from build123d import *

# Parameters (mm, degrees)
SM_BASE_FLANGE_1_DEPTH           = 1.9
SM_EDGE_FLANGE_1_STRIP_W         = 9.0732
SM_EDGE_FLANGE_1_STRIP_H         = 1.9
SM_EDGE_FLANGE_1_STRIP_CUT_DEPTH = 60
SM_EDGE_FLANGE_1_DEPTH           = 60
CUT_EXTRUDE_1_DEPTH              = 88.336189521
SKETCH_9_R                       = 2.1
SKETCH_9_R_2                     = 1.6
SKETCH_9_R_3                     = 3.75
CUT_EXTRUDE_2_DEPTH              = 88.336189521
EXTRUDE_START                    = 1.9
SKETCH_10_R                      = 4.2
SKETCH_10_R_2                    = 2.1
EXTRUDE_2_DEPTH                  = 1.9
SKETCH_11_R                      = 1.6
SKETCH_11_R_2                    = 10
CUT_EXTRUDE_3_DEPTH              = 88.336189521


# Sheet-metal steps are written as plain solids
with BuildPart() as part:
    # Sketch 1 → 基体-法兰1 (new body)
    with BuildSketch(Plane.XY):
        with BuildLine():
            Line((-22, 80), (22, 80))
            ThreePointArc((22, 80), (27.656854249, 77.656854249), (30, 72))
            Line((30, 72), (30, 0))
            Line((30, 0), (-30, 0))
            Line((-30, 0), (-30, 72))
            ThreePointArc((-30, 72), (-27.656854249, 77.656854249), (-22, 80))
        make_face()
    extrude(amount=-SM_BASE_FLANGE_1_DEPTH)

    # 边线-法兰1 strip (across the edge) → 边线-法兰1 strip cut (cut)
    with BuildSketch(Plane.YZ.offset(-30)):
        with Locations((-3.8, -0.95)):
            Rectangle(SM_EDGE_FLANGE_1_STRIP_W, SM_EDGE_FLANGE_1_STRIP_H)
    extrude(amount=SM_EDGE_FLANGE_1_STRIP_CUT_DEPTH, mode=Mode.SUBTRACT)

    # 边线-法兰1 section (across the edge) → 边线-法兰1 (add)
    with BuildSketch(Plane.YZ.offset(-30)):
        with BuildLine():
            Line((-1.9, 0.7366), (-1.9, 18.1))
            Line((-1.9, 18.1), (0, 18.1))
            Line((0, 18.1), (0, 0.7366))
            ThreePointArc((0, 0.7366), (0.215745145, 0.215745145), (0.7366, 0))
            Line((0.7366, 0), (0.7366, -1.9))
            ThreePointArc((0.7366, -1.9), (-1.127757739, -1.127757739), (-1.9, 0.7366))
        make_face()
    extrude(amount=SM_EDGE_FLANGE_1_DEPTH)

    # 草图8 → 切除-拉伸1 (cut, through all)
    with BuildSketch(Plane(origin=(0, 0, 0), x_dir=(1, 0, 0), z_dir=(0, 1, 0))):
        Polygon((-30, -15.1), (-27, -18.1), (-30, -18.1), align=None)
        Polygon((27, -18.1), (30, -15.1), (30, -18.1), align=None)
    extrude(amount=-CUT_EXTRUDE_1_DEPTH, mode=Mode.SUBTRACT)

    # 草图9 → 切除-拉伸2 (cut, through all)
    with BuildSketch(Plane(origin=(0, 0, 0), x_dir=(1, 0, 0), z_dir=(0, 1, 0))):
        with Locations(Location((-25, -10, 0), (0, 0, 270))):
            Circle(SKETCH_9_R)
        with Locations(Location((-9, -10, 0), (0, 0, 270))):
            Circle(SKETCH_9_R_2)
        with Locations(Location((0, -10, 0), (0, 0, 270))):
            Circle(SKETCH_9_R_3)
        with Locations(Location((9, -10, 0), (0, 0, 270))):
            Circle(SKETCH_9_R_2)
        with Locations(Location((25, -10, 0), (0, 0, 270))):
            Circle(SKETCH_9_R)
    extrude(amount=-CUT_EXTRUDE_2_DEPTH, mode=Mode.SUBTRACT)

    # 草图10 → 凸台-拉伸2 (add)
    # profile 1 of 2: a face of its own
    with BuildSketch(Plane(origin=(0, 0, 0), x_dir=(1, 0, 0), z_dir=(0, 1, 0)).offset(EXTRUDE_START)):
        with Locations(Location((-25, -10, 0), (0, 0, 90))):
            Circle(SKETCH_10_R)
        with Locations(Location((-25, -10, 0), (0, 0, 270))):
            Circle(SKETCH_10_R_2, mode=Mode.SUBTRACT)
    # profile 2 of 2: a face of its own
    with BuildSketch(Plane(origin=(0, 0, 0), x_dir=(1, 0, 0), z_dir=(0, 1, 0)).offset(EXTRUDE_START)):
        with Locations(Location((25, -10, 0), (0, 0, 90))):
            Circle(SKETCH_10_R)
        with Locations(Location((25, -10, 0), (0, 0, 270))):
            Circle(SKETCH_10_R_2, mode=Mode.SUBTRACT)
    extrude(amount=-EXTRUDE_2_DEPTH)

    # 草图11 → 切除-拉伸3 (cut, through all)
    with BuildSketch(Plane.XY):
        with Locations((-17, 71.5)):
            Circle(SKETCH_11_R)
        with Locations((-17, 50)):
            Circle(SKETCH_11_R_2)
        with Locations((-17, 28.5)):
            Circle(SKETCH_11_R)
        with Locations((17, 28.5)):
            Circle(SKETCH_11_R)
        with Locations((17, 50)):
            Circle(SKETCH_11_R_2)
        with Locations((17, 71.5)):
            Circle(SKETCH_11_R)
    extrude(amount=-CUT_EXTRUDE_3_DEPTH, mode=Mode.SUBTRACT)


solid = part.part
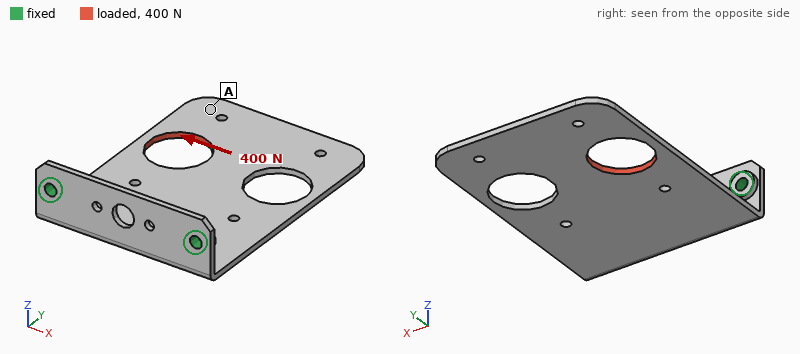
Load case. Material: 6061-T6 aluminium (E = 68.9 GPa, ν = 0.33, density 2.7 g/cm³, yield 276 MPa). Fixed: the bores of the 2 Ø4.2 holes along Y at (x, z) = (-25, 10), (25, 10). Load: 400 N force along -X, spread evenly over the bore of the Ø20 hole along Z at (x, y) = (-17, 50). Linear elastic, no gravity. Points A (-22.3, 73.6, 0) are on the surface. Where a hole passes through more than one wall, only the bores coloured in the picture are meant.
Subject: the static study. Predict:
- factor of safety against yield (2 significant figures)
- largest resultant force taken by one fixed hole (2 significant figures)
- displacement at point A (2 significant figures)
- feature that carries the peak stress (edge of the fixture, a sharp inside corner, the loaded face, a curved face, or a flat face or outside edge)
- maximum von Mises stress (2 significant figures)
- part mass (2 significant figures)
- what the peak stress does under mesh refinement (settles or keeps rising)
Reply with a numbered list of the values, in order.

1. 0.98
2. 470 N
3. 0.43 mm
4. a flat face or outside edge
5. 280 MPa
6. 27 g
7. settles
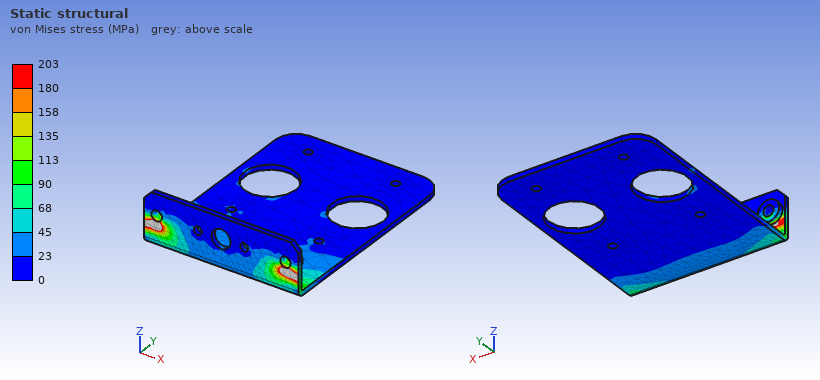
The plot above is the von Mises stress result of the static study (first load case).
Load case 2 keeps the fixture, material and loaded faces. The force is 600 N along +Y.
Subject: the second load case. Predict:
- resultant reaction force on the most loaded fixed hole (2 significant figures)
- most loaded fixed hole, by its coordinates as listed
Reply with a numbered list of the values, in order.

1. 510 N
2. (-25, 10)
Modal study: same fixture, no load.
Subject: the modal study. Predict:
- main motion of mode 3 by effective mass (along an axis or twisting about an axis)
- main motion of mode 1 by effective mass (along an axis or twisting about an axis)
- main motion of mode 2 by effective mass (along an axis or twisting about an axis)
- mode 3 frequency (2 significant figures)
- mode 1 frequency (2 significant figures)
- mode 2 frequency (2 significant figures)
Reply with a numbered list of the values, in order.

1. along Z
2. along Z
3. twisting about Y
4. 1100 Hz
5. 210 Hz
6. 710 Hz
